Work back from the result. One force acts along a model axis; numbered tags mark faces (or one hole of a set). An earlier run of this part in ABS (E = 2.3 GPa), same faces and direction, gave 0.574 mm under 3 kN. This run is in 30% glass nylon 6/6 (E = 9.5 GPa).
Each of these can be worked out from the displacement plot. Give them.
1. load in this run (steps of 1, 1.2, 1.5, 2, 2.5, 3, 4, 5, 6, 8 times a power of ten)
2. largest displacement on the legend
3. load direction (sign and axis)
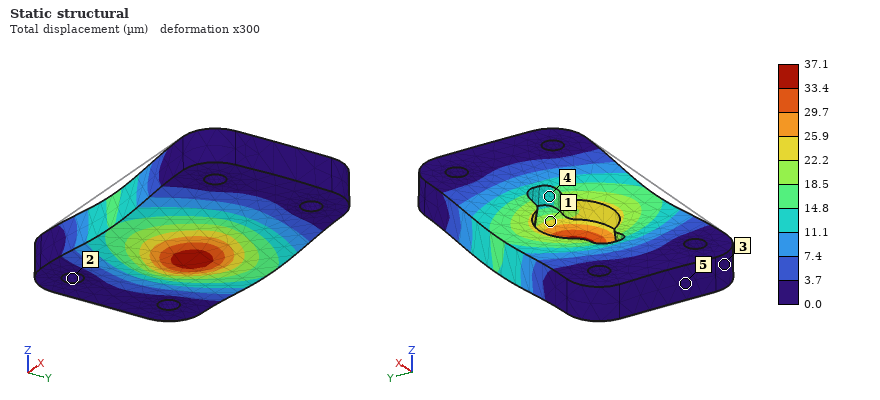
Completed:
800 N
37.1 µm
-Z
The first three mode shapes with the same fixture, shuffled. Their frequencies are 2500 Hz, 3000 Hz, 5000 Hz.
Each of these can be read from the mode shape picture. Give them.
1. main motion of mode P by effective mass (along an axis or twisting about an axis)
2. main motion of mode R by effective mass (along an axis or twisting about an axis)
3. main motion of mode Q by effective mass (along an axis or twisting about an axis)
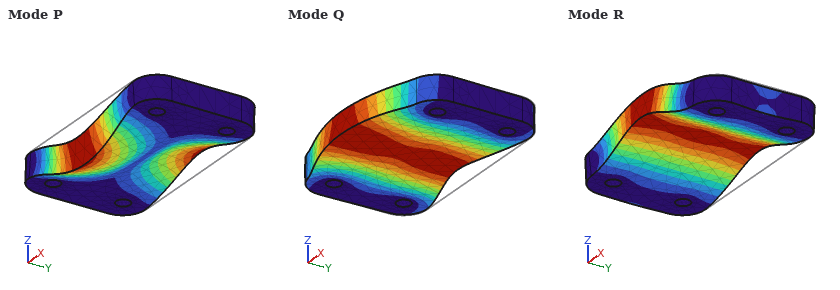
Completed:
twisting about X
along Z
along Y
